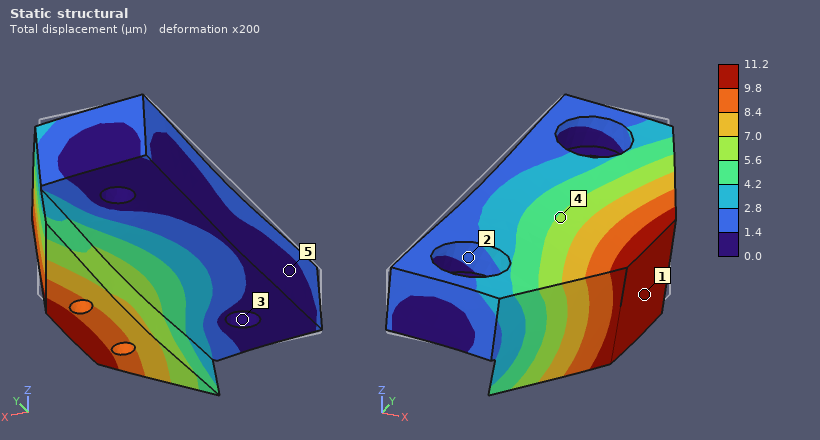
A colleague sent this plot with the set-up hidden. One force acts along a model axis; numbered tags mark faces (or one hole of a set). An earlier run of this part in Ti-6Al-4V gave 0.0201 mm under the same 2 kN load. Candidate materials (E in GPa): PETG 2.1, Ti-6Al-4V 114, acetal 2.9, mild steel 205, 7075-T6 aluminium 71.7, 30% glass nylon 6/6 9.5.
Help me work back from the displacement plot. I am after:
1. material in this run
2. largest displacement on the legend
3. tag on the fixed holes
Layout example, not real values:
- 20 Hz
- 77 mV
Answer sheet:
- mild steel
- 11.2 µm
- 3
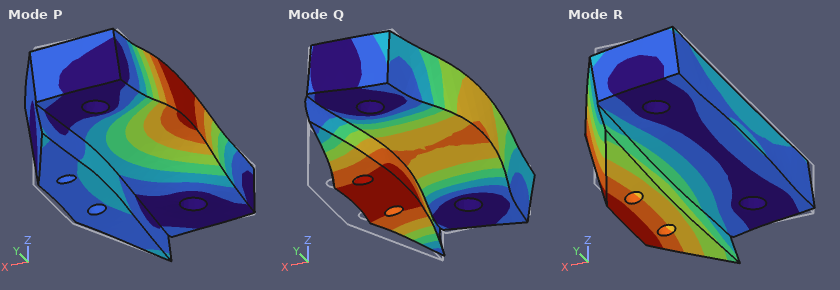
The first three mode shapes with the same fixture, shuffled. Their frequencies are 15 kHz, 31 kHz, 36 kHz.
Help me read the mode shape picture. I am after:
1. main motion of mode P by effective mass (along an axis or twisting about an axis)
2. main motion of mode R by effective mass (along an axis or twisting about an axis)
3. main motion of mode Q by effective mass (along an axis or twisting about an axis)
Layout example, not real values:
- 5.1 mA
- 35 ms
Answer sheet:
- along Z
- along Z
- along X
